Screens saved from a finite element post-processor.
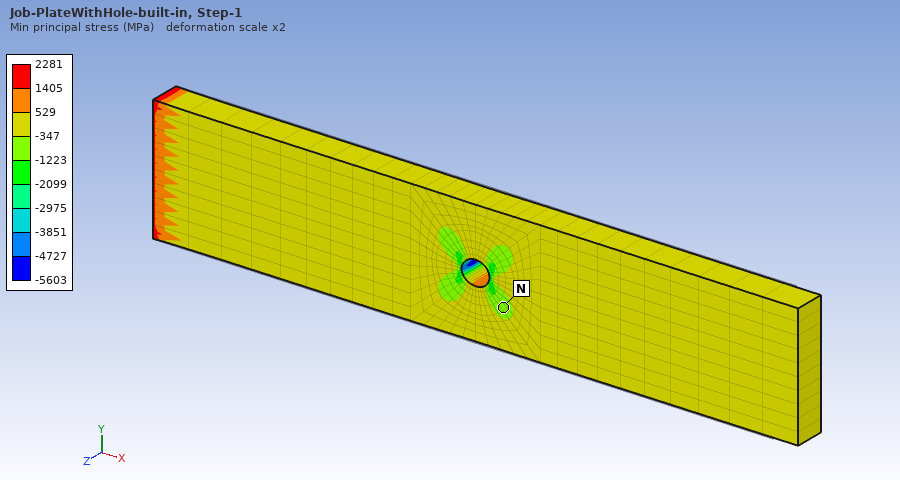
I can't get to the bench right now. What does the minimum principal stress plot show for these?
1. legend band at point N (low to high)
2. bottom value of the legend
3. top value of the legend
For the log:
-1223 to -347 MPa
-5603 MPa
2281 MPa
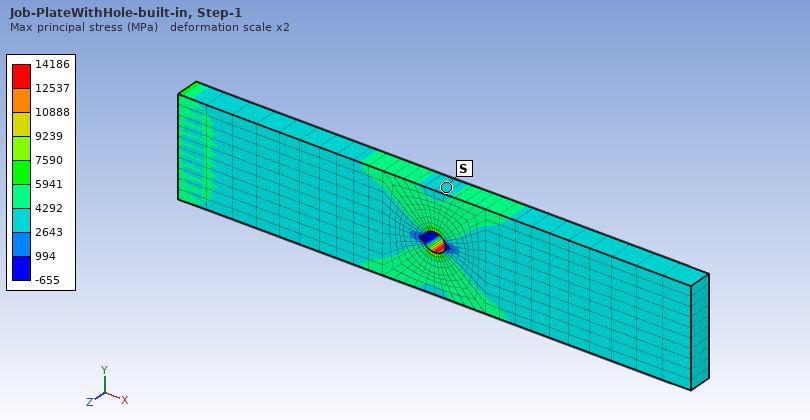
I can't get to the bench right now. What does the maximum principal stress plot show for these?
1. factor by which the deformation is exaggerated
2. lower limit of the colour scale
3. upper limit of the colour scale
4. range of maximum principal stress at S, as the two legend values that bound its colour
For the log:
2
-655 MPa
14186 MPa
2643 to 4292 MPa
